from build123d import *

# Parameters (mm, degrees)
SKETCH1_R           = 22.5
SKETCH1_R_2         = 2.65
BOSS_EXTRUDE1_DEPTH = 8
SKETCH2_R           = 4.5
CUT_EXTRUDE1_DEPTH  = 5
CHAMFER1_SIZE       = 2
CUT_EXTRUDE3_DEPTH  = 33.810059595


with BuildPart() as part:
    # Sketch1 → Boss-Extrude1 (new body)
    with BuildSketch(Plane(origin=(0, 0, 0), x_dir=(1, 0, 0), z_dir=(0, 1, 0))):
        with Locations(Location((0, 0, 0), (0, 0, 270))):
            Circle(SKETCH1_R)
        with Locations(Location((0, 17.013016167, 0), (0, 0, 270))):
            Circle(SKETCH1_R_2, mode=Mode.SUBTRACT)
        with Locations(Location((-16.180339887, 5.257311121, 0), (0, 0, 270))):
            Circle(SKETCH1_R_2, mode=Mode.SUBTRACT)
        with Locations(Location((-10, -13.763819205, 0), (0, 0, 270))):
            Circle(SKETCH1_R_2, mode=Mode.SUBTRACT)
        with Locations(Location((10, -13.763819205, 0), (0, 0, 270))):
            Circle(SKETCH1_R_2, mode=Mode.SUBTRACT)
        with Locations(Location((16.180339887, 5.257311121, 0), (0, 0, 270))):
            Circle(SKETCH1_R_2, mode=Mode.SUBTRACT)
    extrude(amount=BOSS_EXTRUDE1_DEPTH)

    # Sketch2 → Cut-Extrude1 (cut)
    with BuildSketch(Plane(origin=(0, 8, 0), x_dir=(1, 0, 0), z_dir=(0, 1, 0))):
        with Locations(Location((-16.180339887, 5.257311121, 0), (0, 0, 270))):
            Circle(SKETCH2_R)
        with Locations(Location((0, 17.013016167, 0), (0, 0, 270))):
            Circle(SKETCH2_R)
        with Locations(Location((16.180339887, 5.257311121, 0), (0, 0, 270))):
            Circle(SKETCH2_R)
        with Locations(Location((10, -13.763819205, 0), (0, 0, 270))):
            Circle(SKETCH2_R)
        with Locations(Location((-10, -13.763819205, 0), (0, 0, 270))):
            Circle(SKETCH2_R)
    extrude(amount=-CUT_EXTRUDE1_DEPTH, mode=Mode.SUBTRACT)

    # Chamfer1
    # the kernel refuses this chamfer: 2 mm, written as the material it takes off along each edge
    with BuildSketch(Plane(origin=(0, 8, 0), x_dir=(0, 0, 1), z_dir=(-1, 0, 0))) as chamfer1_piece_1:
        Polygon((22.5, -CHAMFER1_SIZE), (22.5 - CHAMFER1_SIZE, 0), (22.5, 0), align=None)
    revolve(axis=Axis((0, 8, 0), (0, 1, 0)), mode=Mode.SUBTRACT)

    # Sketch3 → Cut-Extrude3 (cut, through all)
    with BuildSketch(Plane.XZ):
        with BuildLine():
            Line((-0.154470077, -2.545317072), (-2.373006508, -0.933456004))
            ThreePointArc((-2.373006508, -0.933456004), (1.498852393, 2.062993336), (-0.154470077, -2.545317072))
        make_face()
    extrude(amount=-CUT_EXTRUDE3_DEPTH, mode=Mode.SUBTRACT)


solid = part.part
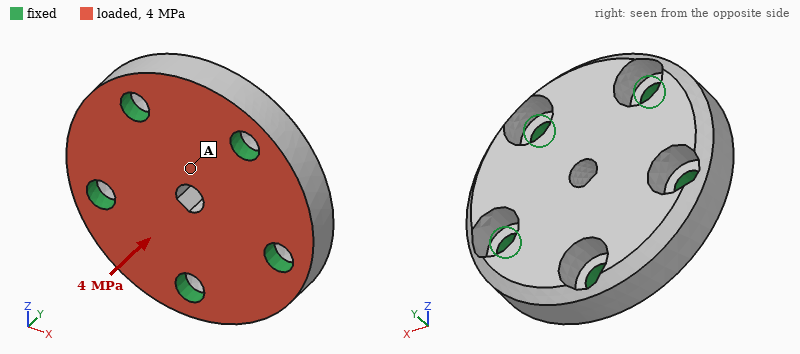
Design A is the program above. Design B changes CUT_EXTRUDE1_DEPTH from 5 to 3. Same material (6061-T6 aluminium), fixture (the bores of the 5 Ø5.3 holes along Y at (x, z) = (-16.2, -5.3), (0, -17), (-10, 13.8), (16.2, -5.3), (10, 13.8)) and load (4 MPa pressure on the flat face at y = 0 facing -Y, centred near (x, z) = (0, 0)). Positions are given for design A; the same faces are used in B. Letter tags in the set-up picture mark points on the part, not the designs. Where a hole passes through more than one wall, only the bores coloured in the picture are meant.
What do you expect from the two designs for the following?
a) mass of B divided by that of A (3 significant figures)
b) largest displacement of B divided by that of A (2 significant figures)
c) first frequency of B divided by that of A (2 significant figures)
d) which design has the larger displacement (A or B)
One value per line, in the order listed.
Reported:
1.04
0.75
1.2
A
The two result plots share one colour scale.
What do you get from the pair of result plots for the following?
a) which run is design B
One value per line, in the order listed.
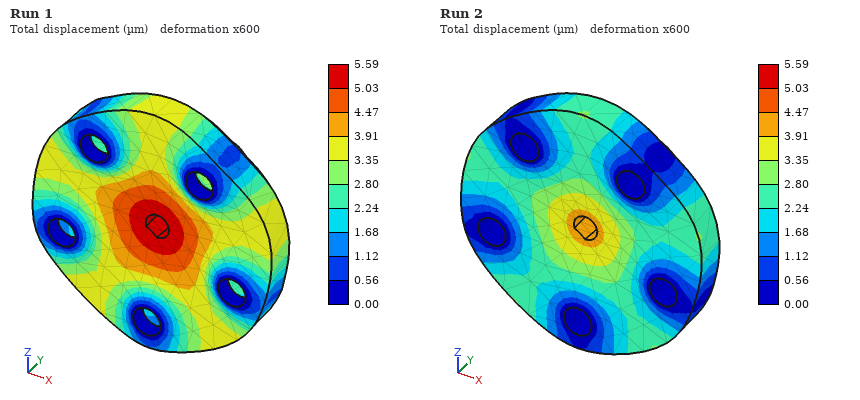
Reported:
Run 2
